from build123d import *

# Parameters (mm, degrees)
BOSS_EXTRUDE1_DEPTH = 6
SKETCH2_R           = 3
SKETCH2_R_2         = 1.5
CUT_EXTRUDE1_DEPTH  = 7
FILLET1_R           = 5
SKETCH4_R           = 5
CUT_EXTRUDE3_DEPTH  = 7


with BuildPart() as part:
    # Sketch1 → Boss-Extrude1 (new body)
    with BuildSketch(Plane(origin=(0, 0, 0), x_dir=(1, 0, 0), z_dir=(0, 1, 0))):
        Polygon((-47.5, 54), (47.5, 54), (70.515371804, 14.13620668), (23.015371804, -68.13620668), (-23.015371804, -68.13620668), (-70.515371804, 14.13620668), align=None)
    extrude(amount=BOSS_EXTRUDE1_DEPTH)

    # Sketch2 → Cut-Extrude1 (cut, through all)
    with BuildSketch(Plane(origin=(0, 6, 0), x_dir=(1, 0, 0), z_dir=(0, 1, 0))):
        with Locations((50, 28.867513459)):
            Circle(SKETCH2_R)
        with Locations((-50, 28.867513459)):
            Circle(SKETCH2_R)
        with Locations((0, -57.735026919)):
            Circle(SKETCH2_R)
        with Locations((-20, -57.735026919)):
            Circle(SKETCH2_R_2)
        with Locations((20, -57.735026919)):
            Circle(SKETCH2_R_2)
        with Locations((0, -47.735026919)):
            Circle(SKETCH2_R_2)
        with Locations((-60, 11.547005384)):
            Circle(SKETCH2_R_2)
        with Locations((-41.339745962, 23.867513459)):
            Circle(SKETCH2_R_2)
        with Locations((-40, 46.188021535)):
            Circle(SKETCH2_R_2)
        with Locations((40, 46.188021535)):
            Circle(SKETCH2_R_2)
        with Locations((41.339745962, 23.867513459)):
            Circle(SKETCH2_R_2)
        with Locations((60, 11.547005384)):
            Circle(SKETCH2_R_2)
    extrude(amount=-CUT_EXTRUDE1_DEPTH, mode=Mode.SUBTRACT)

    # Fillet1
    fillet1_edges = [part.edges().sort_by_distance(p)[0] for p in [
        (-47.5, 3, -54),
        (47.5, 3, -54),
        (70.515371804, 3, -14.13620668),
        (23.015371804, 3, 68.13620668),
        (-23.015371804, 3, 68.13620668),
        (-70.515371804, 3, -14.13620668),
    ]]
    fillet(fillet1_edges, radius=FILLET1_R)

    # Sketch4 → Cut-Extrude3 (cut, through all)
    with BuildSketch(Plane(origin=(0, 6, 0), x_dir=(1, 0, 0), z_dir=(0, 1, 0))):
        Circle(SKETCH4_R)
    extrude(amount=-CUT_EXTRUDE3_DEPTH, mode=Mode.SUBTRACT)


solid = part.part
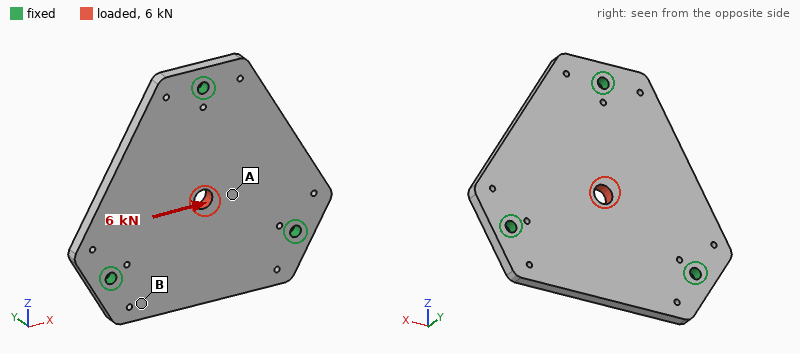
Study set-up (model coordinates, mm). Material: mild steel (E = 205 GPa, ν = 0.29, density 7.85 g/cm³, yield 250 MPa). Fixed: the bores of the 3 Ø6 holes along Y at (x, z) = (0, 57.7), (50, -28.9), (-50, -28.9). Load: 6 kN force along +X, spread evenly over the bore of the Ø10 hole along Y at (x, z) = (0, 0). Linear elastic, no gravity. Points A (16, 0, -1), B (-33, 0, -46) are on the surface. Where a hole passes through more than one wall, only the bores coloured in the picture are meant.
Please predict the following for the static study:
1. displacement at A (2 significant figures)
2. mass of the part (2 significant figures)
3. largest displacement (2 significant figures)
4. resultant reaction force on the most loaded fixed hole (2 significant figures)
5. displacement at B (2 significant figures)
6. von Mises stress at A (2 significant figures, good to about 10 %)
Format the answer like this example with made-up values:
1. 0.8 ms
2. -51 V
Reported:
1. 4.0 µm
2. 570 g
3. 5.6 µm
4. 2.3 kN
5. 1.2 µm
6. 20 MPa
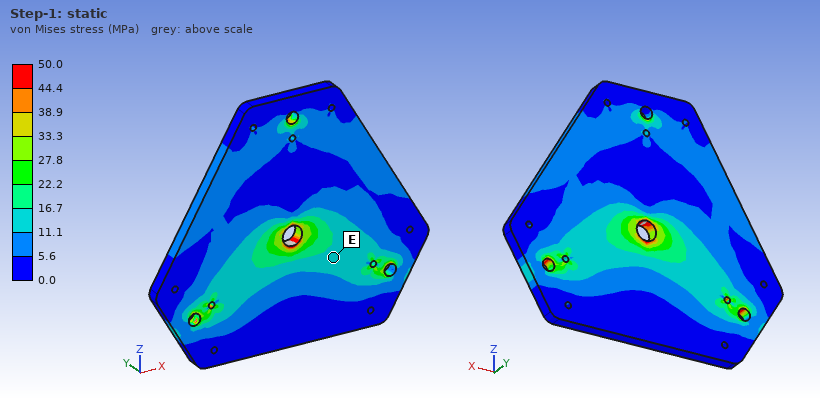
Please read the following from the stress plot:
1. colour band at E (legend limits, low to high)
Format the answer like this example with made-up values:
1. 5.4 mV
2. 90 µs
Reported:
1. 11.1 to 16.7 MPa
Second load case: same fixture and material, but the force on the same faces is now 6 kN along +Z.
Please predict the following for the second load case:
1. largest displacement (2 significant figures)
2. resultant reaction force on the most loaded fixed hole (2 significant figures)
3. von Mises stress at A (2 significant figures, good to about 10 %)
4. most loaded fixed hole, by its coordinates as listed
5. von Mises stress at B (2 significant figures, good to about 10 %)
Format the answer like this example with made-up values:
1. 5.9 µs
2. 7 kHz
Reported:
1. 5.6 µm
2. 2.5 kN
3. 8.5 MPa
4. (0, 57.7)
5. 5.3 MPa
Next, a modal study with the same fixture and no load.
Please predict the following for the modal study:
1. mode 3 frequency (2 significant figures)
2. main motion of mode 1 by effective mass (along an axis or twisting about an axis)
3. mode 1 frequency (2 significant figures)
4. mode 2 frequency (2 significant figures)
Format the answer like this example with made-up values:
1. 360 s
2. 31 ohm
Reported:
1. 2900 Hz
2. along Y
3. 2600 Hz
4. 2900 Hz
